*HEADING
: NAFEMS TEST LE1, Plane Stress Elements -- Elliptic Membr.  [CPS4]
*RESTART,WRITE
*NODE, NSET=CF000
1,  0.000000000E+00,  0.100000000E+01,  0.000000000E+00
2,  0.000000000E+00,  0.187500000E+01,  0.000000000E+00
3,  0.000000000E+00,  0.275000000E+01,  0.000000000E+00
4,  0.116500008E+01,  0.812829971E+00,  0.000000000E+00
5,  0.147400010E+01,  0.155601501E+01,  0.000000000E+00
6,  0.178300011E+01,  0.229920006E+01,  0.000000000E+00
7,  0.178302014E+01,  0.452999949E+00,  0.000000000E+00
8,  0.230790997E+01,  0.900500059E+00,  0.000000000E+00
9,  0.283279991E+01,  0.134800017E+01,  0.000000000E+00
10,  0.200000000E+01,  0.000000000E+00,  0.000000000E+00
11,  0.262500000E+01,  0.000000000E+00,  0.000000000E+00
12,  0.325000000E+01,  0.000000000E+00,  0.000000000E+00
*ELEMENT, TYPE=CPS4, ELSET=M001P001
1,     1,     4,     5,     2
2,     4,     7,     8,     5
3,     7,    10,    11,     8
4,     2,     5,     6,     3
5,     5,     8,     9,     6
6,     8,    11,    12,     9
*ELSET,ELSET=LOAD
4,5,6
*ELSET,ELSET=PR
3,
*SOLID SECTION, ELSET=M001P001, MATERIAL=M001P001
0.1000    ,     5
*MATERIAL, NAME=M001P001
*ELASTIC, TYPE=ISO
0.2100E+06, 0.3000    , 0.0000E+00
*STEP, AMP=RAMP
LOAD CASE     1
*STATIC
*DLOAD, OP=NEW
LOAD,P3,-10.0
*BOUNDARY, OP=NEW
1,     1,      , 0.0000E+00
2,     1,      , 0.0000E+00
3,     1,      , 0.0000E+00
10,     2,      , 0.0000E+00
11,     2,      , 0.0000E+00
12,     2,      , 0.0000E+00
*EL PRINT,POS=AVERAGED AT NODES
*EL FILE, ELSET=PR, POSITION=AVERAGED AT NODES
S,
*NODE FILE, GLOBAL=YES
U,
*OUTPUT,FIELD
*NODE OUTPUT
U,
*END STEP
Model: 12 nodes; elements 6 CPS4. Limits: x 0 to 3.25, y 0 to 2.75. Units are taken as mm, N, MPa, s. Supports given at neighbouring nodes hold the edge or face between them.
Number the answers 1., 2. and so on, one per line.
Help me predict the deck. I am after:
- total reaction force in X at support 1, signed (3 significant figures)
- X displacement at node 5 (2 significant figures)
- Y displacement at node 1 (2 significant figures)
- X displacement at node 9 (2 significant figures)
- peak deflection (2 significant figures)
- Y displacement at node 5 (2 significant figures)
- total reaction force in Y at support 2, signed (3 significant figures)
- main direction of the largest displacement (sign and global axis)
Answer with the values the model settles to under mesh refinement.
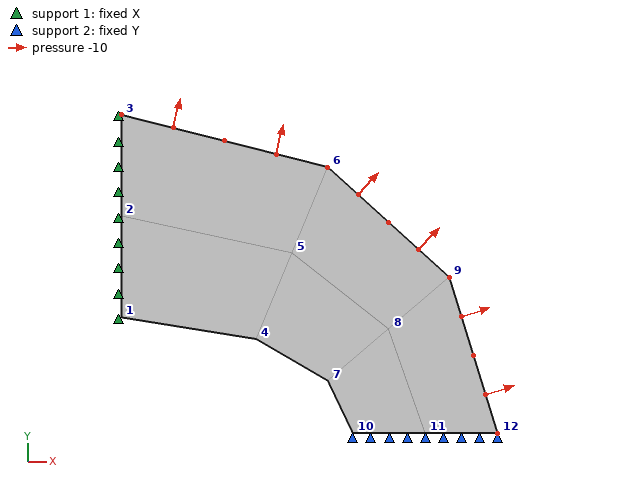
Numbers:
1. -2.75 N
2. 7.2e-05 mm
3. 5.5e-04 mm
4. 7.4e-05 mm
5. 5.6e-04 mm
6. 3.6e-04 mm
7. -3.25 N
8. +Y
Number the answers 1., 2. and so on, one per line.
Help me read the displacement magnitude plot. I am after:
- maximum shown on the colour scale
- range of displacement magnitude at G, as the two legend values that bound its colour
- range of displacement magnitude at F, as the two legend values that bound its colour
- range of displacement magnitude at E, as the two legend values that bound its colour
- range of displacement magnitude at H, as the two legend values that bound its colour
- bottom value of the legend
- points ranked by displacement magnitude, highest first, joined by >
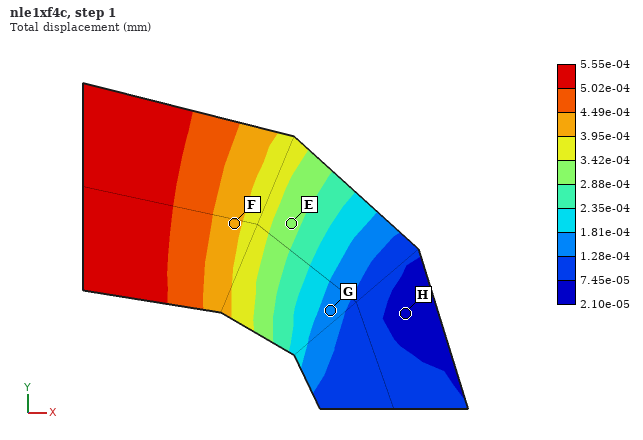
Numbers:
1. 5.55e-04 mm
2. 1.28e-04 to 1.81e-04 mm
3. 3.95e-04 to 4.49e-04 mm
4. 2.88e-04 to 3.42e-04 mm
5. 2.10e-05 to 7.45e-05 mm
6. 2.10e-05 mm
7. F > E > G > H
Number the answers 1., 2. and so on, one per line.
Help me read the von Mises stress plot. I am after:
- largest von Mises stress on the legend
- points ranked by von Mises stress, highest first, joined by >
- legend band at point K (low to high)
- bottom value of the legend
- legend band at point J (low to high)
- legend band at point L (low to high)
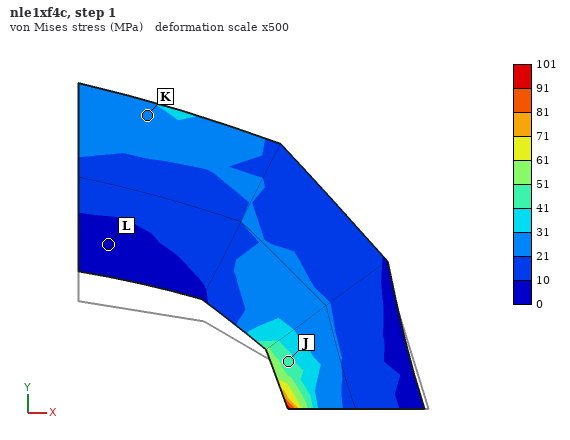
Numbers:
1. 101 MPa
2. J > K > L
3. 21 to 31 MPa
4. 0 MPa
5. 41 to 51 MPa
6. 0 to 10 MPa
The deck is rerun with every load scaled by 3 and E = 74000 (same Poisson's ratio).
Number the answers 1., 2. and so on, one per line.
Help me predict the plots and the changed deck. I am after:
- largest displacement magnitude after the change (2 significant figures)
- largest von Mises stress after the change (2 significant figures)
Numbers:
1. 0.0047 mm
2. 300 MPa
